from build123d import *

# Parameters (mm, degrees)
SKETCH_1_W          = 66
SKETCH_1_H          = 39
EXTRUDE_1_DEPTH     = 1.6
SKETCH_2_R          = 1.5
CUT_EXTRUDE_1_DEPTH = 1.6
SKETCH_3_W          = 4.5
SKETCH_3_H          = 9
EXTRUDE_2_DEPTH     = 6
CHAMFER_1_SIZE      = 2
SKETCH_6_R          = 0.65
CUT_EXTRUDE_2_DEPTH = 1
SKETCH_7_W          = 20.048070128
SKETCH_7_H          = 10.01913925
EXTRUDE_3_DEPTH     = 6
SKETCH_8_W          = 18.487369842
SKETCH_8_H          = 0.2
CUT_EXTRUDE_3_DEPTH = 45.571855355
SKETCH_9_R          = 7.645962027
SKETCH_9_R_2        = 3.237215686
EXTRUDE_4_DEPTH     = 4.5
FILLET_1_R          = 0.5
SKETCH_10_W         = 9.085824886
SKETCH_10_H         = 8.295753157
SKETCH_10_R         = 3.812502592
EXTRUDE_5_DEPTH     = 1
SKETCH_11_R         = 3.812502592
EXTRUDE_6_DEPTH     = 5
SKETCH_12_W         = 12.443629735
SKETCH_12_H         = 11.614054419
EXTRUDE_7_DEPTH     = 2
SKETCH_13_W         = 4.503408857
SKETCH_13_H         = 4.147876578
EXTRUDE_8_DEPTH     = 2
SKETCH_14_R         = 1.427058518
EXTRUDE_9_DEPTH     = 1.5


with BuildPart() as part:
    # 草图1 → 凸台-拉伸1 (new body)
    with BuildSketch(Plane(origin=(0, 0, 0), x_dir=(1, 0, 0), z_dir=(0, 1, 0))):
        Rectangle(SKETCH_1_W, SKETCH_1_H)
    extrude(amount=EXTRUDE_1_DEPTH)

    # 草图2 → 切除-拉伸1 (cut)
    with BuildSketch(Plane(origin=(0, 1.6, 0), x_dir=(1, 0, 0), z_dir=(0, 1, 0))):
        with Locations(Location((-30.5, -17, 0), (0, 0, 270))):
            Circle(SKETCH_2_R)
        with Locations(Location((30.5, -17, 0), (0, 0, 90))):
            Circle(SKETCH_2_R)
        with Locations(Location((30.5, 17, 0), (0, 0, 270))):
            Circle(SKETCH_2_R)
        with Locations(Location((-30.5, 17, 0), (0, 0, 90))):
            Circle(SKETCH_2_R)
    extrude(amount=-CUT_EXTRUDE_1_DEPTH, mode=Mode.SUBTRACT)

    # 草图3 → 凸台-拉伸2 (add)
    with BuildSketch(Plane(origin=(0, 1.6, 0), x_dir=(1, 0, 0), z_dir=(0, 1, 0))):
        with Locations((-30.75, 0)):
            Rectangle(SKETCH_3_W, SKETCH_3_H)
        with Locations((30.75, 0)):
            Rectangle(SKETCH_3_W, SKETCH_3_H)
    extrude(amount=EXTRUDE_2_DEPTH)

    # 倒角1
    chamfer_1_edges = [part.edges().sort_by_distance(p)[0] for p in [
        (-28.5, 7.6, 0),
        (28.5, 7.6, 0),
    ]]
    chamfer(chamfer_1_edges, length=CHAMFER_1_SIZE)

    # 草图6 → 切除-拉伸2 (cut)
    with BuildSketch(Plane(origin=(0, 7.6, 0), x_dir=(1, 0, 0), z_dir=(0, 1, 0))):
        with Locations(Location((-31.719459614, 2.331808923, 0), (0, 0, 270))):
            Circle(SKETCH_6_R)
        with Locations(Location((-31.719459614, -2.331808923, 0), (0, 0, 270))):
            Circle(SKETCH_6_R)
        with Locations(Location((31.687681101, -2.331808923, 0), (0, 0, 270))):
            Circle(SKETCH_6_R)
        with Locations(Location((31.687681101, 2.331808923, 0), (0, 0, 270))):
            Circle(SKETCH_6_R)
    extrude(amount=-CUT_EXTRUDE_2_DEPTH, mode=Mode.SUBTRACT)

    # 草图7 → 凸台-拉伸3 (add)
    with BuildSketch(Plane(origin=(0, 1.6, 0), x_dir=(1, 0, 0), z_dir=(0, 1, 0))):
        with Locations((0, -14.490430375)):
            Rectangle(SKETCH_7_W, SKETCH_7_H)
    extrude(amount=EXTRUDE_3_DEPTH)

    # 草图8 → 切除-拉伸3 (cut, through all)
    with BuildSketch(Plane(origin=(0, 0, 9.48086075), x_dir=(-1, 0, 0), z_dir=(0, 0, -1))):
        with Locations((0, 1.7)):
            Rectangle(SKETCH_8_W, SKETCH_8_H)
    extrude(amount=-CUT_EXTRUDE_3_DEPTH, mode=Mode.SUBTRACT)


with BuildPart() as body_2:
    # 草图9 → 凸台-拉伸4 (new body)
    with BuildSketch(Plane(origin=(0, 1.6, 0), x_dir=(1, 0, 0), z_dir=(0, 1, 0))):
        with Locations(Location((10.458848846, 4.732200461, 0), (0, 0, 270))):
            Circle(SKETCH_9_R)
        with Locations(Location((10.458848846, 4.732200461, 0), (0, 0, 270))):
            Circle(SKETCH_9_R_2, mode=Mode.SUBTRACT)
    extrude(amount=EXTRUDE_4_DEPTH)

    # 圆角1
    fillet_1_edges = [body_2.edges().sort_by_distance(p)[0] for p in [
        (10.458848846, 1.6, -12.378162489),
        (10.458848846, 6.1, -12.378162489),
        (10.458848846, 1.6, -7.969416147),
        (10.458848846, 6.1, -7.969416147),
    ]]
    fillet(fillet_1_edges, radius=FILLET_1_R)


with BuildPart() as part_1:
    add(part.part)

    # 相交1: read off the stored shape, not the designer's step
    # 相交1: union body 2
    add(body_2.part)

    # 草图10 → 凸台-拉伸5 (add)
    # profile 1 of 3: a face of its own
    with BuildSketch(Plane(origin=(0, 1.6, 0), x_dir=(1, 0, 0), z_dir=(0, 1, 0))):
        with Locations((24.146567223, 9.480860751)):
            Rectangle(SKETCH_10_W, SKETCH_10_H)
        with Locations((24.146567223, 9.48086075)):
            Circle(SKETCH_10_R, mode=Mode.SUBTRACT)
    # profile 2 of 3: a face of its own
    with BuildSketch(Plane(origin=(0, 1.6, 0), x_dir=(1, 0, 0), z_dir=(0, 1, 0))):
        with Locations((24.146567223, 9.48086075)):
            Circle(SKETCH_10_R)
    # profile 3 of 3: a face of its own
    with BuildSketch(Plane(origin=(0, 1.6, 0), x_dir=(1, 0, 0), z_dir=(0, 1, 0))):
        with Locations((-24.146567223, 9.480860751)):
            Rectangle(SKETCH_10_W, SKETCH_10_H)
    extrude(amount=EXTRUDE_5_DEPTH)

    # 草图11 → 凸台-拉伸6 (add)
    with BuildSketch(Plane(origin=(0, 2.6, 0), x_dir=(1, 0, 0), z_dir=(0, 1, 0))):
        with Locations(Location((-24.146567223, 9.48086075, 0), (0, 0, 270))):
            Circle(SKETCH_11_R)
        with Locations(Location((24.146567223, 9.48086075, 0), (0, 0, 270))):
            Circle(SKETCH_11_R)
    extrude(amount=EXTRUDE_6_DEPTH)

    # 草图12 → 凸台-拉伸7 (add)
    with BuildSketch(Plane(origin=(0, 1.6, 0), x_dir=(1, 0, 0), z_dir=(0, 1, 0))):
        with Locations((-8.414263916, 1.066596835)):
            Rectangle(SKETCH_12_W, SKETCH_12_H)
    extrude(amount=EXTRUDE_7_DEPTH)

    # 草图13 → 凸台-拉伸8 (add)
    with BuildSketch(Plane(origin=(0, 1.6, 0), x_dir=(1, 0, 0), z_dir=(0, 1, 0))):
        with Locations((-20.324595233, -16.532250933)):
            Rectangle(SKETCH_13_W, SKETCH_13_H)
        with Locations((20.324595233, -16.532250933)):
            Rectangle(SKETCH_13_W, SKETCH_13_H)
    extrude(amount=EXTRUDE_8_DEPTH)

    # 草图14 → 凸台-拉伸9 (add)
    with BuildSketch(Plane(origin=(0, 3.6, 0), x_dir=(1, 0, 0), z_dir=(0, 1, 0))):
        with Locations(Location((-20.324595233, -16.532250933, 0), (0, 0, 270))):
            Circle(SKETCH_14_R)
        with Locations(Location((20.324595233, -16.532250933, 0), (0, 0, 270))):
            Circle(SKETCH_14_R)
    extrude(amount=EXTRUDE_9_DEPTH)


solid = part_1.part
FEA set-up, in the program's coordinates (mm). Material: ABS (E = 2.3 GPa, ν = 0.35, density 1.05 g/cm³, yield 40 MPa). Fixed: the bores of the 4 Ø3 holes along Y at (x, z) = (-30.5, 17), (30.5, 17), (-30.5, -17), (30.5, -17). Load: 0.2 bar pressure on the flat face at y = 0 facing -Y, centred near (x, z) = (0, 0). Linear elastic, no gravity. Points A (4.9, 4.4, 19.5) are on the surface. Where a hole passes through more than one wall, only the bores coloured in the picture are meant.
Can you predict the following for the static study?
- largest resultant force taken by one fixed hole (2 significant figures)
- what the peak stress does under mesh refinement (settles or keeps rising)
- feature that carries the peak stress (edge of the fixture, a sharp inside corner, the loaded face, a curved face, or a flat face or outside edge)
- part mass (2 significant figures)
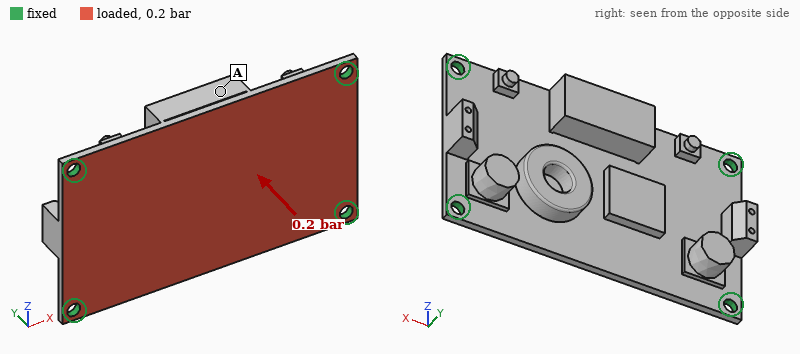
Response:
16 N
keeps rising
edge of the fixture
7.7 g
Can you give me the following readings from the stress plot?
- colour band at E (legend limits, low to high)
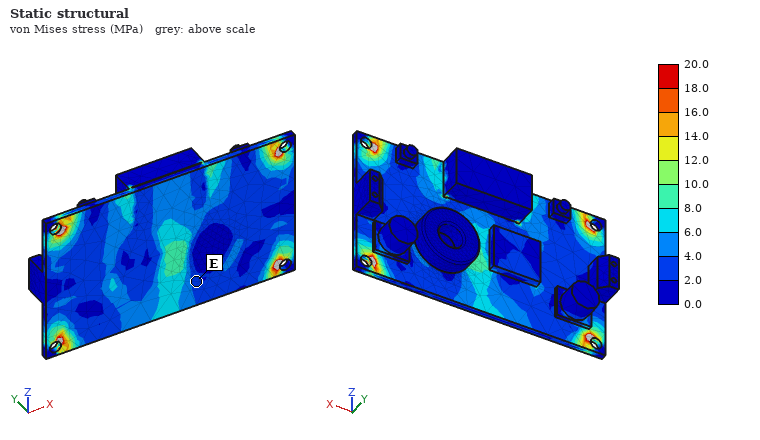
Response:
2.0 to 4.0 MPa
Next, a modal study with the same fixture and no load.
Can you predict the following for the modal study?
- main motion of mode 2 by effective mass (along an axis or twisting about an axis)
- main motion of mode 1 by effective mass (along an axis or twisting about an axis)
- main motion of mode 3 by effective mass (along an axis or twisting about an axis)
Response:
twisting about X
along Y
twisting about Z
